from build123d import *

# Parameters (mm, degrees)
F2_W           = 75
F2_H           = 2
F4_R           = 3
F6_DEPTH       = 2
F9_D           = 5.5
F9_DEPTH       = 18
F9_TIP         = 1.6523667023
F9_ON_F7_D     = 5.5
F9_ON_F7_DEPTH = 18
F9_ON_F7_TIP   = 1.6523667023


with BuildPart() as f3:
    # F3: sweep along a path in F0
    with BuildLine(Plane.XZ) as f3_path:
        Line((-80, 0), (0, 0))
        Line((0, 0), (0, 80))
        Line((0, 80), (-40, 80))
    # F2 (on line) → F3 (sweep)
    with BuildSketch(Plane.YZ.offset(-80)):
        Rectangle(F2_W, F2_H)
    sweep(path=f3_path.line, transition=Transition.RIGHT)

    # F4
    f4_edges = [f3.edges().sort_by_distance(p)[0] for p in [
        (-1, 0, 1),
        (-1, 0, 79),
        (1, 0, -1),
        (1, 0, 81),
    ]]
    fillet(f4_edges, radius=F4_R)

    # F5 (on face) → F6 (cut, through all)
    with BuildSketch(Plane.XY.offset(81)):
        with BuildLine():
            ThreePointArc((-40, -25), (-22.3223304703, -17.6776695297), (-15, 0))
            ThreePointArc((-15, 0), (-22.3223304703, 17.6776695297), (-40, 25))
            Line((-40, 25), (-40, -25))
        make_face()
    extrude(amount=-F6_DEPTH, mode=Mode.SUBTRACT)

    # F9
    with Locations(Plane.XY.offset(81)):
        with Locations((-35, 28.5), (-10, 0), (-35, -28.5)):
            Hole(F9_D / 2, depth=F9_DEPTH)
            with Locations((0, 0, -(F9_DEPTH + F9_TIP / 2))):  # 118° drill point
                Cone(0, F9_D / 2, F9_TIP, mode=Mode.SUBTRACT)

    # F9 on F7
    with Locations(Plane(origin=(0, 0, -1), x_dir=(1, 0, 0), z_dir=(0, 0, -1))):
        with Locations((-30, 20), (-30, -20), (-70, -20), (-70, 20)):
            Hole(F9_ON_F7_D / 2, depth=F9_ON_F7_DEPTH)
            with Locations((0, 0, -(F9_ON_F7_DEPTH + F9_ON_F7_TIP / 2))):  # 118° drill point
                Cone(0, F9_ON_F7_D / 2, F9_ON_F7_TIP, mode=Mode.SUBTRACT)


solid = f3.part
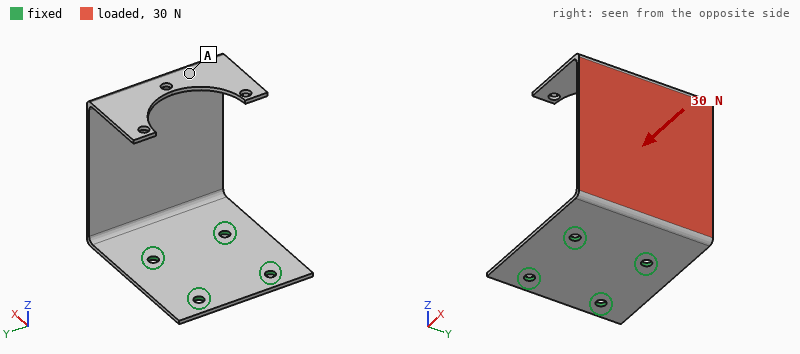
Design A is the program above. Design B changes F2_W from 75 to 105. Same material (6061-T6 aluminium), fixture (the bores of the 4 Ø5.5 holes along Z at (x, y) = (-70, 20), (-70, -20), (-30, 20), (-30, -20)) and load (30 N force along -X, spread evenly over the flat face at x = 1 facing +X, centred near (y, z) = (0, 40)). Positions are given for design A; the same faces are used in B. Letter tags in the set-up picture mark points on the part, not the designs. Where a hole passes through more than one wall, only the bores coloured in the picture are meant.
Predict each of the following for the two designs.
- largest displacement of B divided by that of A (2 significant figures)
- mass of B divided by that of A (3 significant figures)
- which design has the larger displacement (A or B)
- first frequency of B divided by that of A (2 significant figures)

0.74
1.43
A
0.94
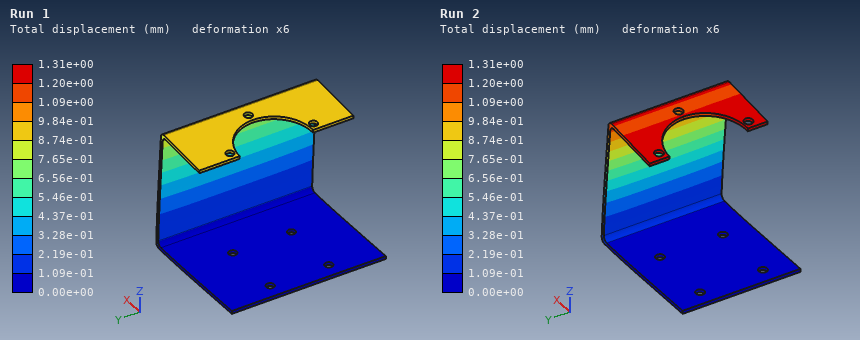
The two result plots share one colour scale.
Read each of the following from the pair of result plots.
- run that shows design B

Run 1
